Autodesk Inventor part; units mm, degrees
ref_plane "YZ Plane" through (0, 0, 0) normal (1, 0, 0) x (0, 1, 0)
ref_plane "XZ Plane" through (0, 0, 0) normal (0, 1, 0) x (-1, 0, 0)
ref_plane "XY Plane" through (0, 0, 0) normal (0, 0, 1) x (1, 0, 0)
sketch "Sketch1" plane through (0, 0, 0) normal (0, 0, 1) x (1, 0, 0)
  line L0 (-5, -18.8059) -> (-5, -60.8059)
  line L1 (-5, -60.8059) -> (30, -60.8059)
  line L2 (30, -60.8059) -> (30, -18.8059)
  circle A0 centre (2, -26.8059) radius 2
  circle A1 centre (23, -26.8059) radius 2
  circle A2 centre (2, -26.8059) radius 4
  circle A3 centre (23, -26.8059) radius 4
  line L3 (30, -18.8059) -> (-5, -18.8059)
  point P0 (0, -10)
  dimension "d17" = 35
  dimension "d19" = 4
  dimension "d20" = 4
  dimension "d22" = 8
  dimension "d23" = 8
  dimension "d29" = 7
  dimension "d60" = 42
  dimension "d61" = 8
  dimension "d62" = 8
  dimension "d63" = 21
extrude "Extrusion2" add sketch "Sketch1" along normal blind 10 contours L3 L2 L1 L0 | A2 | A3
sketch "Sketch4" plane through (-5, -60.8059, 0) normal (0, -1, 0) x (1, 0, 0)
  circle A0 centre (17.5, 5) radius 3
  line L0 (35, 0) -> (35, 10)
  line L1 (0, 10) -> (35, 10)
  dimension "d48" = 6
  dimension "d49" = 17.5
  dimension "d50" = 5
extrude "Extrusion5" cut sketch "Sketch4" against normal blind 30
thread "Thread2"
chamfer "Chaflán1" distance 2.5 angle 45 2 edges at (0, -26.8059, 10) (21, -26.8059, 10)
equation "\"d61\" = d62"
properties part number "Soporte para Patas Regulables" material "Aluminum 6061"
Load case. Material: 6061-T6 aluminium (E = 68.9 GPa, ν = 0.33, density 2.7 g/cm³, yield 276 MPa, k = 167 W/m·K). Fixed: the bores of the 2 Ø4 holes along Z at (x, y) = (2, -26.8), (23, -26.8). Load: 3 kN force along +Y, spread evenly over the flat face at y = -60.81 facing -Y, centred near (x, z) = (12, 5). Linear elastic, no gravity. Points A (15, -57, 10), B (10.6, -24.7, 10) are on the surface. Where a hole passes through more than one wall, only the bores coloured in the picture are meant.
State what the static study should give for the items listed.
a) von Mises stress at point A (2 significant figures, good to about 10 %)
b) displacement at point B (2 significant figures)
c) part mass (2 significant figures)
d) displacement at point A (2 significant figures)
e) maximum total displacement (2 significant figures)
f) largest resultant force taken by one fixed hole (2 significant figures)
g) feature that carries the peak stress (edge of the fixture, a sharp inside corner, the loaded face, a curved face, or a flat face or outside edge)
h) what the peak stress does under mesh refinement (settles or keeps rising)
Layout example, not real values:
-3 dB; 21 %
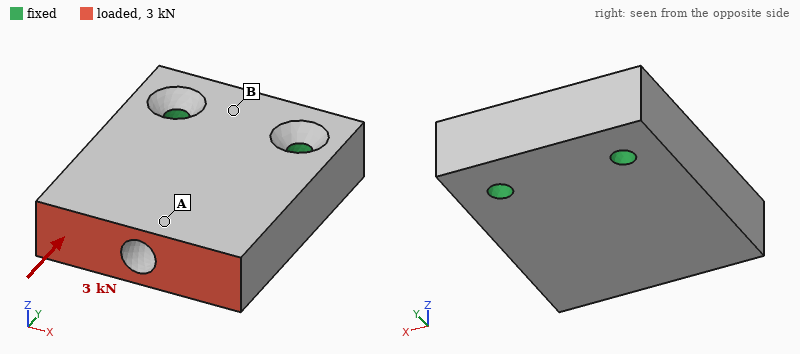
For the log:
9.4 MPa; 1.6 µm; 36 g; 6.3 µm; 7.1 µm; 1.5 kN; edge of the fixture; keeps rising
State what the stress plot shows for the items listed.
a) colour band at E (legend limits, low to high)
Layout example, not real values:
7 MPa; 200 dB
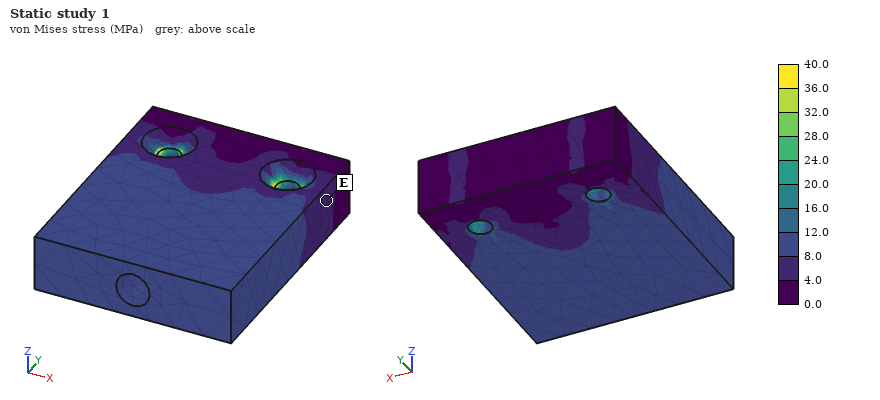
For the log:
4.0 to 8.0 MPa
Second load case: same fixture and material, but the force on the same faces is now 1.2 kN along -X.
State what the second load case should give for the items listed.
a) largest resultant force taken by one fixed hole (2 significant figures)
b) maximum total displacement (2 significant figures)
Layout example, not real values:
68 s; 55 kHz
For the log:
1.8 kN; 19 µm
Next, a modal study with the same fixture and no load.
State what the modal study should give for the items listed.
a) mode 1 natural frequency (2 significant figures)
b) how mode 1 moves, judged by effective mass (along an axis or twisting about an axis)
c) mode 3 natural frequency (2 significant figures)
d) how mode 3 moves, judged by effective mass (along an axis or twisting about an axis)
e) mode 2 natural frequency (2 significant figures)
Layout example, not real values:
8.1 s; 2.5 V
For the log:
5700 Hz; along Z; 14 kHz; along X; 12 kHz
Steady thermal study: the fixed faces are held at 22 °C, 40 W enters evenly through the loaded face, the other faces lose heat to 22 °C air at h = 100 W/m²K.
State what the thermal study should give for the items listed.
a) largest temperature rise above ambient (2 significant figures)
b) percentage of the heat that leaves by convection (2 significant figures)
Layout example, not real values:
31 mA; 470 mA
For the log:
24 K; 12 %
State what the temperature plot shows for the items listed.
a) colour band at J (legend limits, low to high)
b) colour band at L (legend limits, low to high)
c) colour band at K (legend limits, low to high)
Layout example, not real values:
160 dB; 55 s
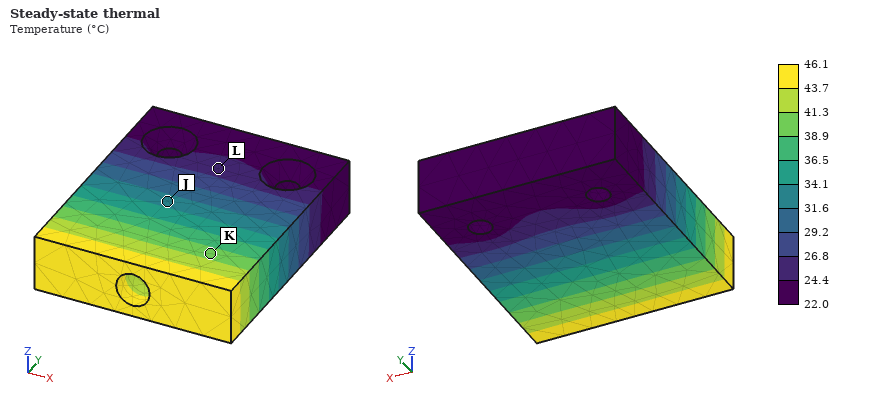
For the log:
31.6 to 34.1 °C; 24.4 to 26.8 °C; 38.9 to 41.3 °C
